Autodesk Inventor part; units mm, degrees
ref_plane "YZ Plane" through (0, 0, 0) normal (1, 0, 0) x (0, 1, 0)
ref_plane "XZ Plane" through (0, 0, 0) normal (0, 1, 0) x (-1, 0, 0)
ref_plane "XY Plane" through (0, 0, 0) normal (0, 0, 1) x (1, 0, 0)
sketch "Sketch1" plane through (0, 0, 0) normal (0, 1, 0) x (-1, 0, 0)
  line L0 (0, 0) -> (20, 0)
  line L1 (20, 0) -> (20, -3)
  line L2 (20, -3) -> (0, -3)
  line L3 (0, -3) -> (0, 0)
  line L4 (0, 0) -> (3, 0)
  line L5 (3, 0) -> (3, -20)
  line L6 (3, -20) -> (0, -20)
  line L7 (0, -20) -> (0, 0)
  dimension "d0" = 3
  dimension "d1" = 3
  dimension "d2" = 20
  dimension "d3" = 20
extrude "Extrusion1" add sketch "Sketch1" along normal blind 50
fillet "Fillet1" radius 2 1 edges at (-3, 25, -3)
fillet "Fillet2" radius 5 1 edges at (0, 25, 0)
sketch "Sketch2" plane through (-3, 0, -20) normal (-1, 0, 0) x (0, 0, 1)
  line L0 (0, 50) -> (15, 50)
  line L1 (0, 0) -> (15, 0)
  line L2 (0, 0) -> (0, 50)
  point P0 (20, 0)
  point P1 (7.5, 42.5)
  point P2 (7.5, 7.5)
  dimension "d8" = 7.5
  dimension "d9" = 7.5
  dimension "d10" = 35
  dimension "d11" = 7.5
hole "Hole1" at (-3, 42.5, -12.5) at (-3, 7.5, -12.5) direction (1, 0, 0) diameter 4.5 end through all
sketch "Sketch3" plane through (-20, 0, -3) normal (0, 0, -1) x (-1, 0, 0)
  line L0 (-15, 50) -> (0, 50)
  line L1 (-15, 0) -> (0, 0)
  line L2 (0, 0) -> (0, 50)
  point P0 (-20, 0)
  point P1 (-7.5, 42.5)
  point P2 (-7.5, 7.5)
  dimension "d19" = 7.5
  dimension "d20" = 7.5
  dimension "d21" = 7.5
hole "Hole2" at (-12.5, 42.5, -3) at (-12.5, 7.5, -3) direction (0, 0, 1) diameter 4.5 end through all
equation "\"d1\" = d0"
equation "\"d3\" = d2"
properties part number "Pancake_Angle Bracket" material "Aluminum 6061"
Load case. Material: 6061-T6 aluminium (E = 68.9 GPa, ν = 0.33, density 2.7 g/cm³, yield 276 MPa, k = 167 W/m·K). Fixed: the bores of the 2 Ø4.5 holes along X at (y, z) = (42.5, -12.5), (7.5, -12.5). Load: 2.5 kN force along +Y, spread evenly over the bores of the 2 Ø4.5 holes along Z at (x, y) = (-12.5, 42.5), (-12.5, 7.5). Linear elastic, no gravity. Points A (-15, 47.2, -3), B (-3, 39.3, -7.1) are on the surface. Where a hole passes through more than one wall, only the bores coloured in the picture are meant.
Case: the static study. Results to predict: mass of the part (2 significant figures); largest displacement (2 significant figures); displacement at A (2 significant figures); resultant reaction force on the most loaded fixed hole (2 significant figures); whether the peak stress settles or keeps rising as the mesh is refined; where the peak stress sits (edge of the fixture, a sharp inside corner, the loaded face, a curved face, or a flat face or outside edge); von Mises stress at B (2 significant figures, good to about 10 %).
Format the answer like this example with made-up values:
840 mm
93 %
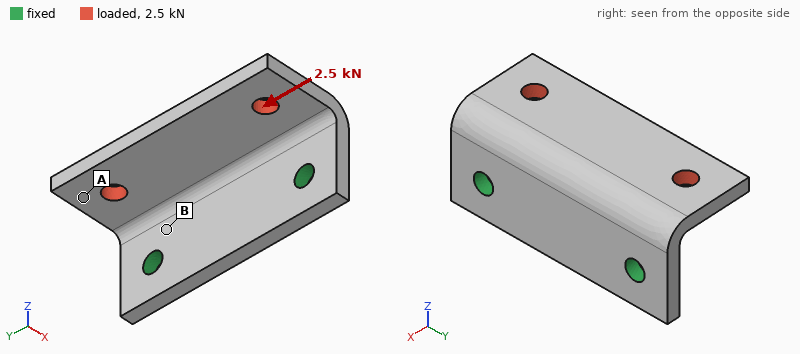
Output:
14 g
0.17 mm
0.13 mm
1.6 kN
keeps rising
edge of the fixture
110 MPa
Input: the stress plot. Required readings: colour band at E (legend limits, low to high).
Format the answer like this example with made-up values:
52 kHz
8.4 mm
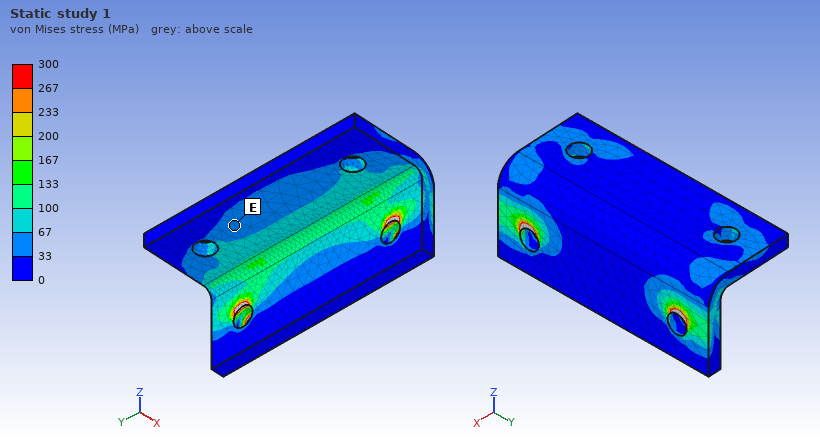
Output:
33 to 67 MPa
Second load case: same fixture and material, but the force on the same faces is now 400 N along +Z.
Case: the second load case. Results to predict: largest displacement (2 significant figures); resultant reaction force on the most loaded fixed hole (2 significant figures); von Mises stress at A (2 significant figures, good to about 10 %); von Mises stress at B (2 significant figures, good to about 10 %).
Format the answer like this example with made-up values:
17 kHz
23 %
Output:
0.16 mm
200 N
14 MPa
65 MPa
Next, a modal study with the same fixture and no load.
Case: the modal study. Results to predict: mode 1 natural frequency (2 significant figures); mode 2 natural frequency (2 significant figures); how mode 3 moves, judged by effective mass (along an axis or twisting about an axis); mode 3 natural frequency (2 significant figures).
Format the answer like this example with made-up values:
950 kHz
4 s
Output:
3800 Hz
6200 Hz
along X
11 kHz
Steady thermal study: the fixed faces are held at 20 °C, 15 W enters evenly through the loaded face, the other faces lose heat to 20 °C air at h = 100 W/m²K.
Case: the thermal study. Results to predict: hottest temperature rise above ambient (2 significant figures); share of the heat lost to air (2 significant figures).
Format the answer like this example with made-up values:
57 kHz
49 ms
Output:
16 K
18 %
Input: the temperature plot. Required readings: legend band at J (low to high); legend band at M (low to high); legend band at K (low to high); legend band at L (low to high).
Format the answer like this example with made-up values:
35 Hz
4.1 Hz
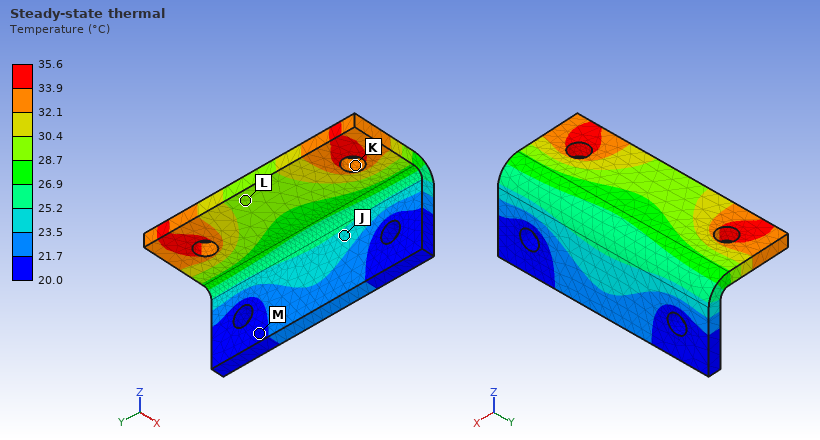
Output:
23.5 to 25.2 °C
20.0 to 21.7 °C
32.1 to 33.9 °C
28.7 to 30.4 °C
